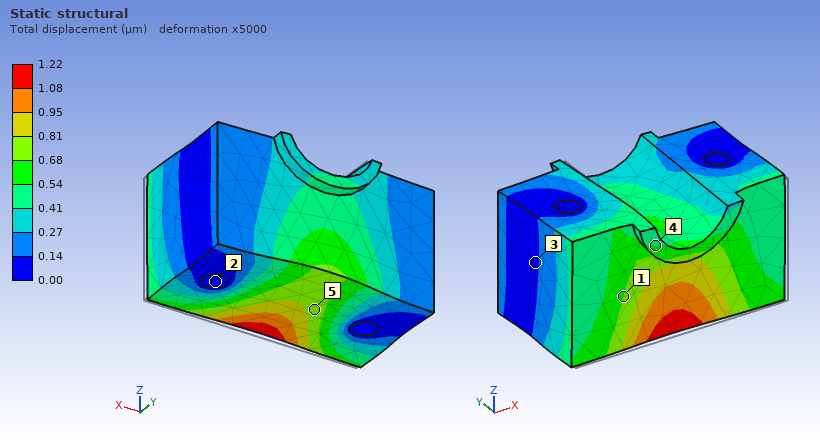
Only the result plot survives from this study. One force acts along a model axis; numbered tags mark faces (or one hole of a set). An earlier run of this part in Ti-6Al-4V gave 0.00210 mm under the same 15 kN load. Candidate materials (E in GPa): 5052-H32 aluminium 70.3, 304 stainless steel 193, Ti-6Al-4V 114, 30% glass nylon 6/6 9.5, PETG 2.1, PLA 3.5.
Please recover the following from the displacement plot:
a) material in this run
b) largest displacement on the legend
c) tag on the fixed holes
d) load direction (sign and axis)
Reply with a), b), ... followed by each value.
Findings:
a) 304 stainless steel
b) 1.22 µm
c) 2
d) +Y
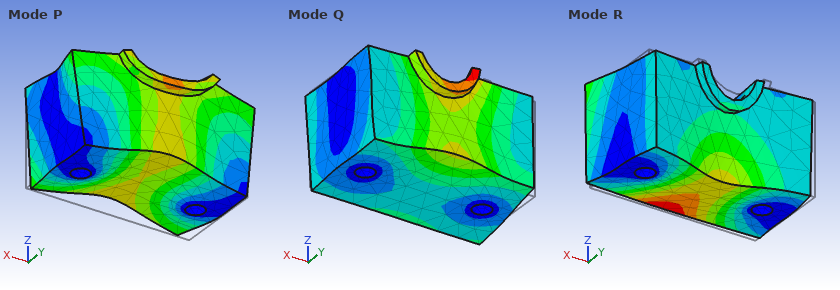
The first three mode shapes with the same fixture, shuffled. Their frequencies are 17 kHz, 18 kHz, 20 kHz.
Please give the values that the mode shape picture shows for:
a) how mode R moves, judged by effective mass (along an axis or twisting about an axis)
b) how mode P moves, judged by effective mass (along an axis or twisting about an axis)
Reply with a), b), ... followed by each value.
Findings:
a) along Y
b) along Z
